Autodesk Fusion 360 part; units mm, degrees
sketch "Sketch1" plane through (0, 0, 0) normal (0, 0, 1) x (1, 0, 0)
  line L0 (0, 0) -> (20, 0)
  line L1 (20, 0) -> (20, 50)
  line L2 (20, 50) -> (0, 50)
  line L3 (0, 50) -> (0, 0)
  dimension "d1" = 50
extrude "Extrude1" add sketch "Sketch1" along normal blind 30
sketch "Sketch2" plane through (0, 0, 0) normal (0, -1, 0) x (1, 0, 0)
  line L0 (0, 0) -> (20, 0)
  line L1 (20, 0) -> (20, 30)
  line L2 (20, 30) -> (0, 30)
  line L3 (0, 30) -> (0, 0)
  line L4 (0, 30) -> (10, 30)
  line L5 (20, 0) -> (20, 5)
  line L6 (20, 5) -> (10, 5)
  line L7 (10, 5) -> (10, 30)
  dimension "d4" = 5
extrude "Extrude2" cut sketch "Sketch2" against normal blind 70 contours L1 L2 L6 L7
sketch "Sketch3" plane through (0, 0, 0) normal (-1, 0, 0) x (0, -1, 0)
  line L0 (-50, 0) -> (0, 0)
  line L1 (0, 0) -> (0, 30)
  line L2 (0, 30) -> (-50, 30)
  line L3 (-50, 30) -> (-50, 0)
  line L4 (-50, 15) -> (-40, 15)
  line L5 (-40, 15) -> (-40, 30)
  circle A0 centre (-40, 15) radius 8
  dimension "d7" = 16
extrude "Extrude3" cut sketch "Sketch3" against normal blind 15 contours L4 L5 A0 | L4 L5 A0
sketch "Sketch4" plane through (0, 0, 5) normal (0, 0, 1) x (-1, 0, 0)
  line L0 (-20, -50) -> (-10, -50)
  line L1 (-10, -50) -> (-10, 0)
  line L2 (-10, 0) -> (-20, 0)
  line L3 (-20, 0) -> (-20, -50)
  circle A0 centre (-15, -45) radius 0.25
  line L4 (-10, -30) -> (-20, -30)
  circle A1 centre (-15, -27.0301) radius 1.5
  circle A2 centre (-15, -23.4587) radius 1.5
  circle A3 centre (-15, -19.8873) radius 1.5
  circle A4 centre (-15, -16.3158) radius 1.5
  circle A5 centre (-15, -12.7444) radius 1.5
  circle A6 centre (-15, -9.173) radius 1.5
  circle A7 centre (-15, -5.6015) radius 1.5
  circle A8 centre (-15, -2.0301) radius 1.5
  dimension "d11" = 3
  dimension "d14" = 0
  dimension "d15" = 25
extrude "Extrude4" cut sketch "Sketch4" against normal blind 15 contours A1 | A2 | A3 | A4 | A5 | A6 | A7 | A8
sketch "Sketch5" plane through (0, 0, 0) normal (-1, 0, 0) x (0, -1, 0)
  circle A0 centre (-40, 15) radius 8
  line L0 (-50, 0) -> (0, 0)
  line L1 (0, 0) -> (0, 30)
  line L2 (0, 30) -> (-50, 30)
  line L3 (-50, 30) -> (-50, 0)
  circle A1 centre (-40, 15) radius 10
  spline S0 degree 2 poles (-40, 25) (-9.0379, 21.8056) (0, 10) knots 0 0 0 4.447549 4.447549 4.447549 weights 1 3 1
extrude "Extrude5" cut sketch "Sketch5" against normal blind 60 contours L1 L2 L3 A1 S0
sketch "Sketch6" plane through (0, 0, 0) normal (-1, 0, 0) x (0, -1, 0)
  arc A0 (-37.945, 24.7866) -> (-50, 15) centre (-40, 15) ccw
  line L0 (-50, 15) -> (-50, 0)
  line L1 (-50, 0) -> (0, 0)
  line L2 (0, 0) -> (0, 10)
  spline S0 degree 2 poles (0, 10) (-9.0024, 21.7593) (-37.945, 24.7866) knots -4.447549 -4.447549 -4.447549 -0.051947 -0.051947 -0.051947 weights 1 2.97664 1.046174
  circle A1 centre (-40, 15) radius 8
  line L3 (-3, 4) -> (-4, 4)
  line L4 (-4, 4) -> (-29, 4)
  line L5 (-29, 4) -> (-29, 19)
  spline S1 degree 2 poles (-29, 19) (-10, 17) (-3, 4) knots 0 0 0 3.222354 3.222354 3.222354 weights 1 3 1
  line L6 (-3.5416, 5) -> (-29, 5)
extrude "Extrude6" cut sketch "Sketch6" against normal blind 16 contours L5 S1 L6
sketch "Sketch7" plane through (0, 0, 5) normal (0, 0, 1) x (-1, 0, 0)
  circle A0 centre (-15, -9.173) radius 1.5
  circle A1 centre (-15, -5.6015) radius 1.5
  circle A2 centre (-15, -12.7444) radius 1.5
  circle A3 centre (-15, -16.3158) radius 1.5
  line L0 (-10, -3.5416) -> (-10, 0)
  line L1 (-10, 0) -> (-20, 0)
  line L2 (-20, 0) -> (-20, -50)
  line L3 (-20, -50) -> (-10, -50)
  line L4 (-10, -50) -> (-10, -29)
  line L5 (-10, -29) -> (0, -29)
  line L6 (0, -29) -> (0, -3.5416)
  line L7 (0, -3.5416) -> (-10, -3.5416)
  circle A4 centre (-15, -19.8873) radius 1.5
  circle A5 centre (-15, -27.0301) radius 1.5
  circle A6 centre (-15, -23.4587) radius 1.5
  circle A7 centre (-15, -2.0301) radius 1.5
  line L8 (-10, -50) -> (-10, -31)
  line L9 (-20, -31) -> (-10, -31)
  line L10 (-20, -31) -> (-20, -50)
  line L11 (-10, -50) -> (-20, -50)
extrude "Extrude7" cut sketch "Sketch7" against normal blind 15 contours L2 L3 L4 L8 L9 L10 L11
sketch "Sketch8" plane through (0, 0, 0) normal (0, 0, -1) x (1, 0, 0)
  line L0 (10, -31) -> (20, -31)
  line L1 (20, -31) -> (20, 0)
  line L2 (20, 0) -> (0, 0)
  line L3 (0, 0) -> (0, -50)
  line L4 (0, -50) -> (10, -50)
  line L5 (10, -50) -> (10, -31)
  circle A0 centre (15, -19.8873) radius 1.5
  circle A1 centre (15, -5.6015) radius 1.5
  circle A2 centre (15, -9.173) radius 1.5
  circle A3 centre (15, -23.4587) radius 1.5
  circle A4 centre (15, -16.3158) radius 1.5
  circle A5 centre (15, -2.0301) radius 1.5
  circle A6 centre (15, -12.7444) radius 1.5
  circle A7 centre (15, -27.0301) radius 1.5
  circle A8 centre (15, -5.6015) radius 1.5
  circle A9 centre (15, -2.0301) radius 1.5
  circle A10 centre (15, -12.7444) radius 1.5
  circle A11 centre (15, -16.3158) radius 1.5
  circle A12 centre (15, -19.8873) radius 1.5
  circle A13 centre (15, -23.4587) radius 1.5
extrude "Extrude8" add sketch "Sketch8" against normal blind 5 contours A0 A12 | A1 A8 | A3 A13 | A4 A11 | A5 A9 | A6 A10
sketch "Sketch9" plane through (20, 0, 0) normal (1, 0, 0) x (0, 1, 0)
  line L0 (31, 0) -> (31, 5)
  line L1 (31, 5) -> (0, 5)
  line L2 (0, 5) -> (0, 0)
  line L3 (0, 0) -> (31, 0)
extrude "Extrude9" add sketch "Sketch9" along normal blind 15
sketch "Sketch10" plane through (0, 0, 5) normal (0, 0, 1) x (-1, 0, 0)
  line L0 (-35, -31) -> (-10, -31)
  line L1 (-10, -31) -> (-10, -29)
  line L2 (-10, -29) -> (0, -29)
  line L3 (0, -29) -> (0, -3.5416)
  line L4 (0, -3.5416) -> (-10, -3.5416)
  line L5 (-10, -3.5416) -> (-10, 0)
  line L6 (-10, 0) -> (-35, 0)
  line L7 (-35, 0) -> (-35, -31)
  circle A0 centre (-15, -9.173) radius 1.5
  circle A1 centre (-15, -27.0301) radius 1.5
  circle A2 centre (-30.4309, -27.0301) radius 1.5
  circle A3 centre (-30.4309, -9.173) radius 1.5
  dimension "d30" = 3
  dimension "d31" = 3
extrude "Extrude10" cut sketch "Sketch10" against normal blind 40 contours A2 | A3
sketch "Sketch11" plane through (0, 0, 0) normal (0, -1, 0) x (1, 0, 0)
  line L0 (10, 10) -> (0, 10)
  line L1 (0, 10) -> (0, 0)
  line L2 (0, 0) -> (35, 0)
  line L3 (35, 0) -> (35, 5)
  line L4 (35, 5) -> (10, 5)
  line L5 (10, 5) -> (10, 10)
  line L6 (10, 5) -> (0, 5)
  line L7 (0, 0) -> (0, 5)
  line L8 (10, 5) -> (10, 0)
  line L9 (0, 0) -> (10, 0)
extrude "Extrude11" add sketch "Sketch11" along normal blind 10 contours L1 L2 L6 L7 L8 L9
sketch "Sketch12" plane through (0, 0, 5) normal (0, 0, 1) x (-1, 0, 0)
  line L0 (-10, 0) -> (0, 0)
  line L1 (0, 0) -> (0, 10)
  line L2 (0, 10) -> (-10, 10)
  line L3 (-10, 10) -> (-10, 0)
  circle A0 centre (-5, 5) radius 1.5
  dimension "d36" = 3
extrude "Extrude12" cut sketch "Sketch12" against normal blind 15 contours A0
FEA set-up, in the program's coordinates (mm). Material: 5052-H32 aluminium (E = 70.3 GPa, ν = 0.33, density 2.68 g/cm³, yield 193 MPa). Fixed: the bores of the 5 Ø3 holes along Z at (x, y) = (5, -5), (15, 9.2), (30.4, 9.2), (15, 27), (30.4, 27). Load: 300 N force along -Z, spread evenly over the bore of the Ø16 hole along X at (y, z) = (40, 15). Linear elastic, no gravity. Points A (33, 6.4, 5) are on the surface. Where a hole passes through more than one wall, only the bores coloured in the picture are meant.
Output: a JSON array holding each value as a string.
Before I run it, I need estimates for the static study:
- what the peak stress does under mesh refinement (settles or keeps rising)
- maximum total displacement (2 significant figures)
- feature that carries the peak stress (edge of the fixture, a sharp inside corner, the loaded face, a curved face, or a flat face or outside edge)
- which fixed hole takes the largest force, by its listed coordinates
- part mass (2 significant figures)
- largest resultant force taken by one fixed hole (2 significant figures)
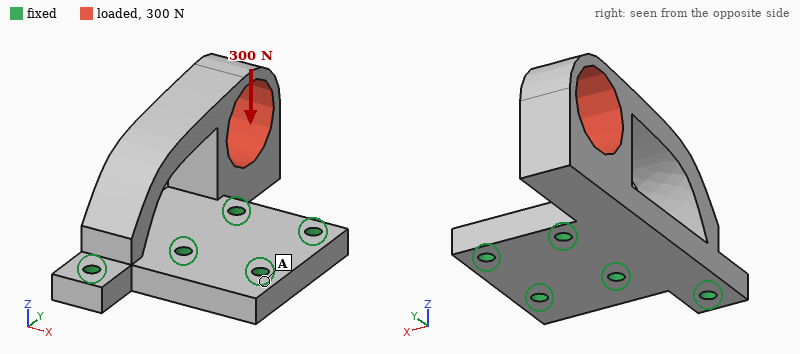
["keeps rising", "54 µm", "edge of the fixture", "(15, 27)", "27 g", "430 N"]
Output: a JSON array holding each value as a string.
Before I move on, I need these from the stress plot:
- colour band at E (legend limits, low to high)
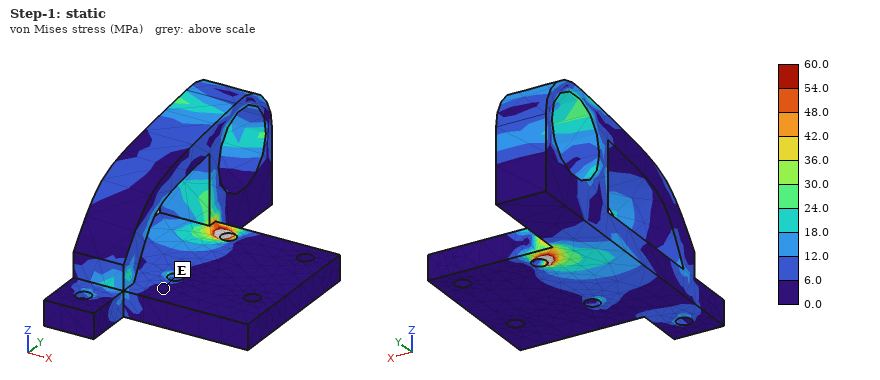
["0.0 to 6.0 MPa"]
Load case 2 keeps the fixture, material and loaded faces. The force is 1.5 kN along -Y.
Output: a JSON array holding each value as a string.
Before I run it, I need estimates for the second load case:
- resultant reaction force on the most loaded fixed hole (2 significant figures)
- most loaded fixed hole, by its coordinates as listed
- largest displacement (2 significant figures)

["900 N", "(5, -5)", "0.11 mm"]
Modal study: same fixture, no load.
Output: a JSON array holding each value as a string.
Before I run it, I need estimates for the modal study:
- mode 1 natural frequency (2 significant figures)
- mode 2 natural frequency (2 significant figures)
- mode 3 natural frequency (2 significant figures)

["4200 Hz", "6500 Hz", "9600 Hz"]
